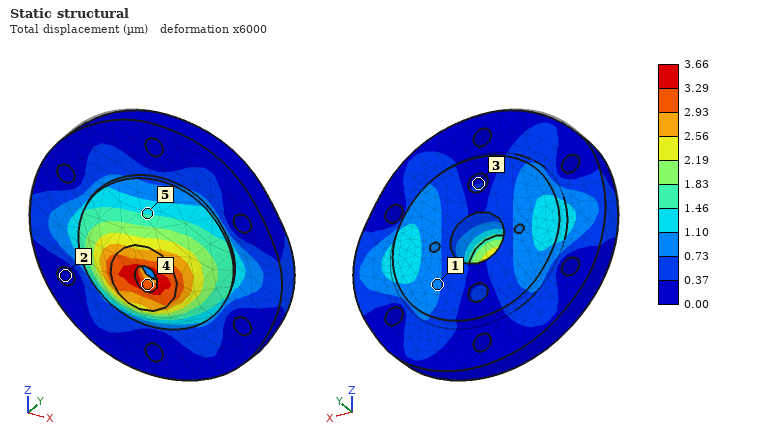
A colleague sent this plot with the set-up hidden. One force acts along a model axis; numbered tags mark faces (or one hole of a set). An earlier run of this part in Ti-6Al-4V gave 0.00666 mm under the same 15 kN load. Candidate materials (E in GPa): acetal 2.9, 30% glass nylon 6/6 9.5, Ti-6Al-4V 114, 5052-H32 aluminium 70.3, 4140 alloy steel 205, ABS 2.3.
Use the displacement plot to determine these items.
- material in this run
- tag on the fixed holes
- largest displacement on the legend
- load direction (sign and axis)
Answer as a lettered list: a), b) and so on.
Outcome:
a) 4140 alloy steel
b) 2
c) 3.66 µm
d) +X
